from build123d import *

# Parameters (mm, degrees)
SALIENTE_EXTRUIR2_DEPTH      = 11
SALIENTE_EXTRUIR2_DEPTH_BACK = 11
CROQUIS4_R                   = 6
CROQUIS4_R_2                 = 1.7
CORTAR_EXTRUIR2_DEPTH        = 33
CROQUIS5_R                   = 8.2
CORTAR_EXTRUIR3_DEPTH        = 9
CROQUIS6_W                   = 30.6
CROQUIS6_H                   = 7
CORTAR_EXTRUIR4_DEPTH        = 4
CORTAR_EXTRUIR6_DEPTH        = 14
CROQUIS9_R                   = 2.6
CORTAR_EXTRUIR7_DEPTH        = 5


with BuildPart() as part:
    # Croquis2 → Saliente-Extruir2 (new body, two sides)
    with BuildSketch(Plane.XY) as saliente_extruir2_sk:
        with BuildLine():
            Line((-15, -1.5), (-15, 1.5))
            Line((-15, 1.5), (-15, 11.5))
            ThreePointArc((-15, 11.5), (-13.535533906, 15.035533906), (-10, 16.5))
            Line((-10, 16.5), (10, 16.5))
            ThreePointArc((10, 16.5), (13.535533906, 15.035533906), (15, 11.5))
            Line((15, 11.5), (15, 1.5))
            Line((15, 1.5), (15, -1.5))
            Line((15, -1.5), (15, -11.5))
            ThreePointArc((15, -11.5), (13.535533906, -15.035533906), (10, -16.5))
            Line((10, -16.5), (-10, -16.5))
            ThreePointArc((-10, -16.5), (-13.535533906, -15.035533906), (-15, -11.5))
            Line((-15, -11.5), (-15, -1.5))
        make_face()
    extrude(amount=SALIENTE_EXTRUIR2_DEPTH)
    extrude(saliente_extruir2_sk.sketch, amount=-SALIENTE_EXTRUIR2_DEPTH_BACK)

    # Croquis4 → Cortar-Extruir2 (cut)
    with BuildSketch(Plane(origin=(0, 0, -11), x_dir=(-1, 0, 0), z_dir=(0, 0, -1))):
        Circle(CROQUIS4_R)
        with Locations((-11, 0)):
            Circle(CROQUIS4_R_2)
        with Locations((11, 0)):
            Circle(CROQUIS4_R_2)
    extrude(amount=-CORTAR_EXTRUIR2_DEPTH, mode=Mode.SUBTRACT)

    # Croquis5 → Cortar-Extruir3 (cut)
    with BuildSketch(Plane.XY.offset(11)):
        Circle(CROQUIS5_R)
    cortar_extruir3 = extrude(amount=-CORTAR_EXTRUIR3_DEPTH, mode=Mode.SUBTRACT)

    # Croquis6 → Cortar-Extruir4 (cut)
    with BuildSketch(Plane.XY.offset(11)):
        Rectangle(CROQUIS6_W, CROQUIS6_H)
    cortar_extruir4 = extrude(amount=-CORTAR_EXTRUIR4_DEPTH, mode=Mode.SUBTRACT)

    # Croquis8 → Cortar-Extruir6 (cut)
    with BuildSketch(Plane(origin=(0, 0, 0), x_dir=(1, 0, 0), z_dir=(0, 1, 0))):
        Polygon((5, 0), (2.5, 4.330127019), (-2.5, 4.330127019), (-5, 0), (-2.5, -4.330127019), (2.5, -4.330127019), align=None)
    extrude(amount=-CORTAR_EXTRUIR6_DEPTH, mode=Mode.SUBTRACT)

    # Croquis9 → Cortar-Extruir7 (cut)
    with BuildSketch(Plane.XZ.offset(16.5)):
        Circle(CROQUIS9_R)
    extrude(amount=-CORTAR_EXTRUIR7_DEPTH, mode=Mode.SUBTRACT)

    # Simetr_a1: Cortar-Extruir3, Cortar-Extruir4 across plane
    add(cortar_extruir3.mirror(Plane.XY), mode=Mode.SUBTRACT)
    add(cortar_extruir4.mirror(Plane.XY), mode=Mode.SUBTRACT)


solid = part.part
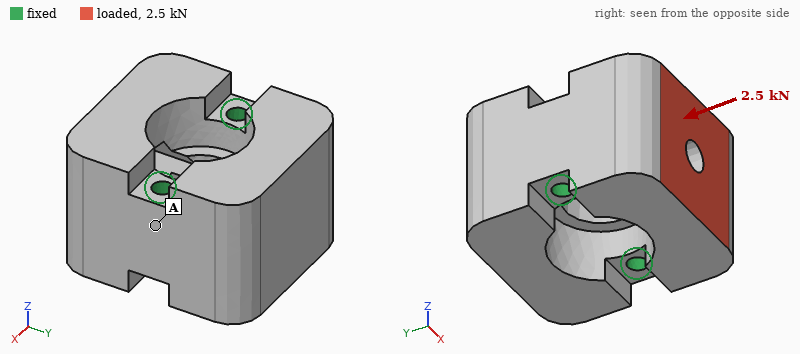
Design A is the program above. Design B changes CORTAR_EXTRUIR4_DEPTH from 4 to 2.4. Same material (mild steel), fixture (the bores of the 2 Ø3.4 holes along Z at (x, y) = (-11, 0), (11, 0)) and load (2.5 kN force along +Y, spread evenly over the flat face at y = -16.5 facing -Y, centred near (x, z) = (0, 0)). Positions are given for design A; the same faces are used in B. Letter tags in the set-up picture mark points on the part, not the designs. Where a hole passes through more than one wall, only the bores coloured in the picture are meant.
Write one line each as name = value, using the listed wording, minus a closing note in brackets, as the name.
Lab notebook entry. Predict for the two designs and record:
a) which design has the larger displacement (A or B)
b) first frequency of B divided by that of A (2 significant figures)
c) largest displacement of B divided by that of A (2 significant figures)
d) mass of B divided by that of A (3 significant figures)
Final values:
which design has the larger displacement = A
first frequency of B divided by that of A = 1.3
largest displacement of B divided by that of A = 0.91
mass of B divided by that of A = 1.02
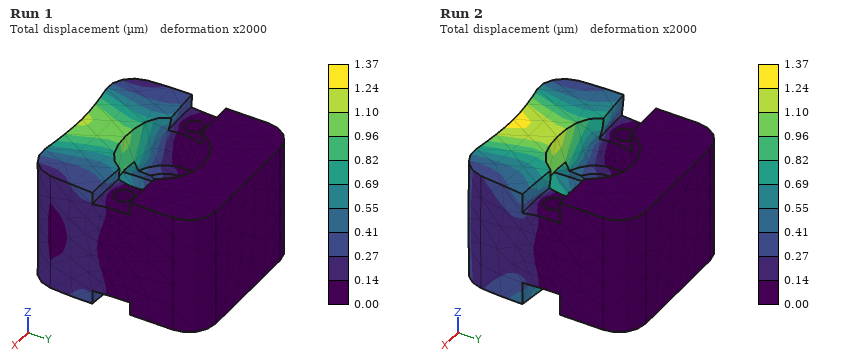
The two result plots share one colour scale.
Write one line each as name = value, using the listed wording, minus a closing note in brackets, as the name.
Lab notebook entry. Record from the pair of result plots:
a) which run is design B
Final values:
which run is design B = Run 1
